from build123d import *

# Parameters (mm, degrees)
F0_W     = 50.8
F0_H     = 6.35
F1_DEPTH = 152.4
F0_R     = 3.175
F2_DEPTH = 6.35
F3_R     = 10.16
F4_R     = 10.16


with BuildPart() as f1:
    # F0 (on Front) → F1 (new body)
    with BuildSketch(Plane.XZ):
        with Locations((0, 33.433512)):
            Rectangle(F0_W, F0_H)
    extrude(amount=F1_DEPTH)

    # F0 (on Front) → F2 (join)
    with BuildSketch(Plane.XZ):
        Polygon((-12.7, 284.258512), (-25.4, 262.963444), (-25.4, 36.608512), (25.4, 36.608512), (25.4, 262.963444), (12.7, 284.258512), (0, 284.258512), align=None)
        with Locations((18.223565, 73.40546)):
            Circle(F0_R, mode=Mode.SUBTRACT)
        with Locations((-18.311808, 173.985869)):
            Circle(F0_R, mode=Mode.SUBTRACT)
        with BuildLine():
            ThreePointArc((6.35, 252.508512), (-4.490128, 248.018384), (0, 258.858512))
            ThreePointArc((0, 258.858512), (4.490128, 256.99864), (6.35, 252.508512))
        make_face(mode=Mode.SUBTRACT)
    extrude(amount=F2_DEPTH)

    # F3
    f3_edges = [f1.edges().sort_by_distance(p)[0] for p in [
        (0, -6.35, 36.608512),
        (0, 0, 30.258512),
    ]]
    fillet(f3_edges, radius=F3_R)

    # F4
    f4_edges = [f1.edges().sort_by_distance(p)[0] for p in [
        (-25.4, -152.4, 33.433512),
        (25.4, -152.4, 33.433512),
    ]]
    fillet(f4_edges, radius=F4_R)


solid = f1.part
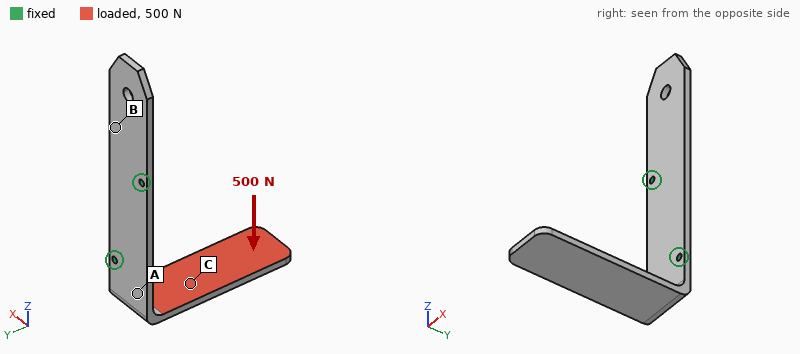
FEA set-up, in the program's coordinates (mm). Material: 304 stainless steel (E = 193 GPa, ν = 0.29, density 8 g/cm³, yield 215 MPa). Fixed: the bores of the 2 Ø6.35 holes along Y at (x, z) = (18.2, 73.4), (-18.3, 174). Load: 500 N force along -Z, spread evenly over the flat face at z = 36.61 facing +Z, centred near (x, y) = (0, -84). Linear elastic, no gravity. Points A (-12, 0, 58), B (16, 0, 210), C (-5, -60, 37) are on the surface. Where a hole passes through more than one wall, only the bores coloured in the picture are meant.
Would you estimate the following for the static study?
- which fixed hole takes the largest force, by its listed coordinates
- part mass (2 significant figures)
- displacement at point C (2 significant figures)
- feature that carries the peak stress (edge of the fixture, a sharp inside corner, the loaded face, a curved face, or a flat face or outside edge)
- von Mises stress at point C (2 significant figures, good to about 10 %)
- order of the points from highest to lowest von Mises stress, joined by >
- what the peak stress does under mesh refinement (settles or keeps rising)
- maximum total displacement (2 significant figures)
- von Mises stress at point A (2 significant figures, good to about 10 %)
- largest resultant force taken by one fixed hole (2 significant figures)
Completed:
(18.2, 73.4)
1.0 kg
0.62 mm
edge of the fixture
45 MPa
A > C > B
keeps rising
2.0 mm
97 MPa
390 N
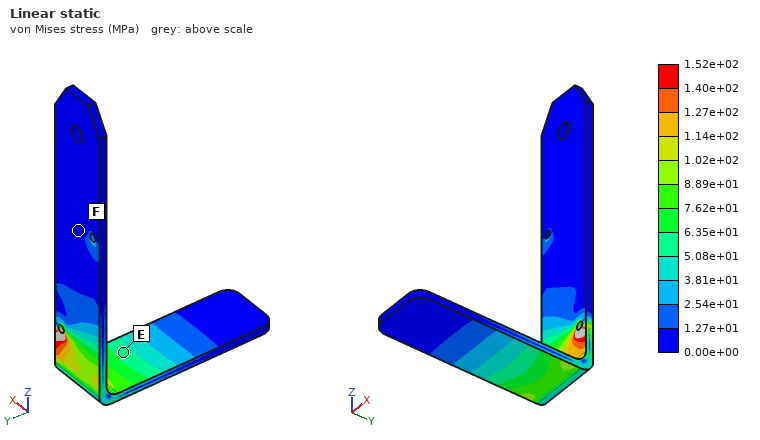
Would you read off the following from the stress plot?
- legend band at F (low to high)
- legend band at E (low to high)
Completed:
0.00e+00 to 1.27e+01 MPa
5.08e+01 to 6.35e+01 MPa
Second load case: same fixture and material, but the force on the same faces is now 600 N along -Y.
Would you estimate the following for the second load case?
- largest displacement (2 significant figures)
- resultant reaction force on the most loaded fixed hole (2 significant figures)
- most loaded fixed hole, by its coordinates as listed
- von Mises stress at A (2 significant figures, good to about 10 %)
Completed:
0.36 mm
670 N
(18.2, 73.4)
28 MPa
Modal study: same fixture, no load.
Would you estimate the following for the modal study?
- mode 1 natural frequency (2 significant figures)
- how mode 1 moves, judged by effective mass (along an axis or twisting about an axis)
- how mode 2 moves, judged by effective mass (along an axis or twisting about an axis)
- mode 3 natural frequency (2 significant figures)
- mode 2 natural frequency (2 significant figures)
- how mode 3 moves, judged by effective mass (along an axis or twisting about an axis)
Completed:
160 Hz
along Z
along X
410 Hz
250 Hz
along Y
